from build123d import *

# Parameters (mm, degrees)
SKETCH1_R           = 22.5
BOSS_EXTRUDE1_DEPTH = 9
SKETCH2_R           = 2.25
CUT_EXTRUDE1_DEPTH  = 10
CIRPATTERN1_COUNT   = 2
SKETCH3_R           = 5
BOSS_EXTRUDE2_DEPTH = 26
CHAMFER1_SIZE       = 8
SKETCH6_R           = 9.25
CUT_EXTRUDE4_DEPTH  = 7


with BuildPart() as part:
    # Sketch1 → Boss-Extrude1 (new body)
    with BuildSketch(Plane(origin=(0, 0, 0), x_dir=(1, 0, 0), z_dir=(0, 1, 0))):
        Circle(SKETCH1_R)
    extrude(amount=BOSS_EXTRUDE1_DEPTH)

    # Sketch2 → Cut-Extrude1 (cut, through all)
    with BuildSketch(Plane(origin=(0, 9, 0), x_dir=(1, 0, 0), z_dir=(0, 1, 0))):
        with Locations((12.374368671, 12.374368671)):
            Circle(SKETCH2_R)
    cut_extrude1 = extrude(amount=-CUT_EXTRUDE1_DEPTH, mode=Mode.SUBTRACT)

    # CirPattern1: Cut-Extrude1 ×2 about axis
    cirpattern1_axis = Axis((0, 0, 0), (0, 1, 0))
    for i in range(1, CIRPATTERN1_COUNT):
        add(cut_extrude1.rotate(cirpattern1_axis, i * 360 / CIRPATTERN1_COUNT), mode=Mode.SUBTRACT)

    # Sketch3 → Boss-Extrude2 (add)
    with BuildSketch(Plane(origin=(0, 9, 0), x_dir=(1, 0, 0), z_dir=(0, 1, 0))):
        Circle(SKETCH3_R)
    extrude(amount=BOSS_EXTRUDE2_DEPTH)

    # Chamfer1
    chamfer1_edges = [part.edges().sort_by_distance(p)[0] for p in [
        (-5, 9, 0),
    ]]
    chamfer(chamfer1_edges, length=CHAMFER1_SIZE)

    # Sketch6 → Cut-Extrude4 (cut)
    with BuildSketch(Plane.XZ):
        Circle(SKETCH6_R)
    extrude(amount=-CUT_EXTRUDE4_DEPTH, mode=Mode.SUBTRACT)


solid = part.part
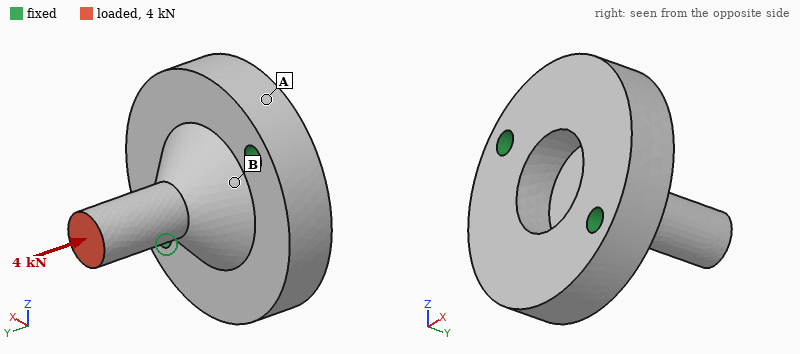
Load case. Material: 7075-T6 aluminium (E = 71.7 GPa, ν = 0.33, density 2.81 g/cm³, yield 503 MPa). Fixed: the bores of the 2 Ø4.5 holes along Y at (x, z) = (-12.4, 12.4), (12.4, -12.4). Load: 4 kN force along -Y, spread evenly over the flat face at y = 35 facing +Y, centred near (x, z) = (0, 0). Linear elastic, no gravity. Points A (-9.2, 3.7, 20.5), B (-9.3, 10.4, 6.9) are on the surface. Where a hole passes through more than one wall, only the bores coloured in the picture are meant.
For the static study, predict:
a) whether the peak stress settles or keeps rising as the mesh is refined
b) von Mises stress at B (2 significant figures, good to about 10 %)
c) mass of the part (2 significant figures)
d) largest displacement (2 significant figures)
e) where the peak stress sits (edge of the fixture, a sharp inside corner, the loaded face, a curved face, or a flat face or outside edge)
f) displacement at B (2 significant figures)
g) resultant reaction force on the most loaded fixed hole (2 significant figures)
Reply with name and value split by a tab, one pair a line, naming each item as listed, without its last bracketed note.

whether the peak stress settles or keeps rising as the mesh is refined	keeps rising
von Mises stress at B	35 MPa
mass of the part	44 g
largest displacement	25 µm
where the peak stress sits	edge of the fixture
displacement at B	5.0 µm
resultant reaction force on the most loaded fixed hole	2.2 kN
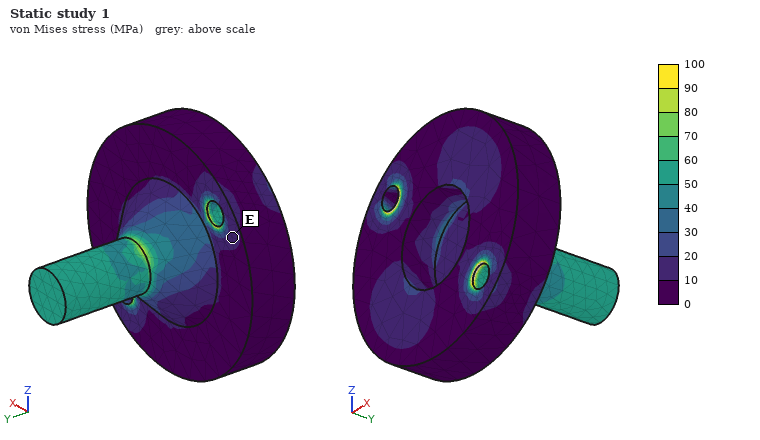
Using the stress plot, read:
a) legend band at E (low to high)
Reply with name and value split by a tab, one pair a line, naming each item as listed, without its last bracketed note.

legend band at E	10 to 20 MPa
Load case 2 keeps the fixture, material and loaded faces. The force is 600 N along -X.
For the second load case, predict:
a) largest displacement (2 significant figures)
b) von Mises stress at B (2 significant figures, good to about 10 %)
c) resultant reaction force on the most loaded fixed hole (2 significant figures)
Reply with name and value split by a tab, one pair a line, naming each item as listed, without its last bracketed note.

largest displacement	75 µm
von Mises stress at B	19 MPa
resultant reaction force on the most loaded fixed hole	530 N
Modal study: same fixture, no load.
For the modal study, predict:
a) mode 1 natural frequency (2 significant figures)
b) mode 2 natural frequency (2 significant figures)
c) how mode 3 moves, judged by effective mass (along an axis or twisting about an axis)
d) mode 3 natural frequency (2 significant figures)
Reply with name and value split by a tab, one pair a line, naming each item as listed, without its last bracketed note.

mode 1 natural frequency	9000 Hz
mode 2 natural frequency	14 kHz
how mode 3 moves, judged by effective mass	along Y
mode 3 natural frequency	16 kHz
